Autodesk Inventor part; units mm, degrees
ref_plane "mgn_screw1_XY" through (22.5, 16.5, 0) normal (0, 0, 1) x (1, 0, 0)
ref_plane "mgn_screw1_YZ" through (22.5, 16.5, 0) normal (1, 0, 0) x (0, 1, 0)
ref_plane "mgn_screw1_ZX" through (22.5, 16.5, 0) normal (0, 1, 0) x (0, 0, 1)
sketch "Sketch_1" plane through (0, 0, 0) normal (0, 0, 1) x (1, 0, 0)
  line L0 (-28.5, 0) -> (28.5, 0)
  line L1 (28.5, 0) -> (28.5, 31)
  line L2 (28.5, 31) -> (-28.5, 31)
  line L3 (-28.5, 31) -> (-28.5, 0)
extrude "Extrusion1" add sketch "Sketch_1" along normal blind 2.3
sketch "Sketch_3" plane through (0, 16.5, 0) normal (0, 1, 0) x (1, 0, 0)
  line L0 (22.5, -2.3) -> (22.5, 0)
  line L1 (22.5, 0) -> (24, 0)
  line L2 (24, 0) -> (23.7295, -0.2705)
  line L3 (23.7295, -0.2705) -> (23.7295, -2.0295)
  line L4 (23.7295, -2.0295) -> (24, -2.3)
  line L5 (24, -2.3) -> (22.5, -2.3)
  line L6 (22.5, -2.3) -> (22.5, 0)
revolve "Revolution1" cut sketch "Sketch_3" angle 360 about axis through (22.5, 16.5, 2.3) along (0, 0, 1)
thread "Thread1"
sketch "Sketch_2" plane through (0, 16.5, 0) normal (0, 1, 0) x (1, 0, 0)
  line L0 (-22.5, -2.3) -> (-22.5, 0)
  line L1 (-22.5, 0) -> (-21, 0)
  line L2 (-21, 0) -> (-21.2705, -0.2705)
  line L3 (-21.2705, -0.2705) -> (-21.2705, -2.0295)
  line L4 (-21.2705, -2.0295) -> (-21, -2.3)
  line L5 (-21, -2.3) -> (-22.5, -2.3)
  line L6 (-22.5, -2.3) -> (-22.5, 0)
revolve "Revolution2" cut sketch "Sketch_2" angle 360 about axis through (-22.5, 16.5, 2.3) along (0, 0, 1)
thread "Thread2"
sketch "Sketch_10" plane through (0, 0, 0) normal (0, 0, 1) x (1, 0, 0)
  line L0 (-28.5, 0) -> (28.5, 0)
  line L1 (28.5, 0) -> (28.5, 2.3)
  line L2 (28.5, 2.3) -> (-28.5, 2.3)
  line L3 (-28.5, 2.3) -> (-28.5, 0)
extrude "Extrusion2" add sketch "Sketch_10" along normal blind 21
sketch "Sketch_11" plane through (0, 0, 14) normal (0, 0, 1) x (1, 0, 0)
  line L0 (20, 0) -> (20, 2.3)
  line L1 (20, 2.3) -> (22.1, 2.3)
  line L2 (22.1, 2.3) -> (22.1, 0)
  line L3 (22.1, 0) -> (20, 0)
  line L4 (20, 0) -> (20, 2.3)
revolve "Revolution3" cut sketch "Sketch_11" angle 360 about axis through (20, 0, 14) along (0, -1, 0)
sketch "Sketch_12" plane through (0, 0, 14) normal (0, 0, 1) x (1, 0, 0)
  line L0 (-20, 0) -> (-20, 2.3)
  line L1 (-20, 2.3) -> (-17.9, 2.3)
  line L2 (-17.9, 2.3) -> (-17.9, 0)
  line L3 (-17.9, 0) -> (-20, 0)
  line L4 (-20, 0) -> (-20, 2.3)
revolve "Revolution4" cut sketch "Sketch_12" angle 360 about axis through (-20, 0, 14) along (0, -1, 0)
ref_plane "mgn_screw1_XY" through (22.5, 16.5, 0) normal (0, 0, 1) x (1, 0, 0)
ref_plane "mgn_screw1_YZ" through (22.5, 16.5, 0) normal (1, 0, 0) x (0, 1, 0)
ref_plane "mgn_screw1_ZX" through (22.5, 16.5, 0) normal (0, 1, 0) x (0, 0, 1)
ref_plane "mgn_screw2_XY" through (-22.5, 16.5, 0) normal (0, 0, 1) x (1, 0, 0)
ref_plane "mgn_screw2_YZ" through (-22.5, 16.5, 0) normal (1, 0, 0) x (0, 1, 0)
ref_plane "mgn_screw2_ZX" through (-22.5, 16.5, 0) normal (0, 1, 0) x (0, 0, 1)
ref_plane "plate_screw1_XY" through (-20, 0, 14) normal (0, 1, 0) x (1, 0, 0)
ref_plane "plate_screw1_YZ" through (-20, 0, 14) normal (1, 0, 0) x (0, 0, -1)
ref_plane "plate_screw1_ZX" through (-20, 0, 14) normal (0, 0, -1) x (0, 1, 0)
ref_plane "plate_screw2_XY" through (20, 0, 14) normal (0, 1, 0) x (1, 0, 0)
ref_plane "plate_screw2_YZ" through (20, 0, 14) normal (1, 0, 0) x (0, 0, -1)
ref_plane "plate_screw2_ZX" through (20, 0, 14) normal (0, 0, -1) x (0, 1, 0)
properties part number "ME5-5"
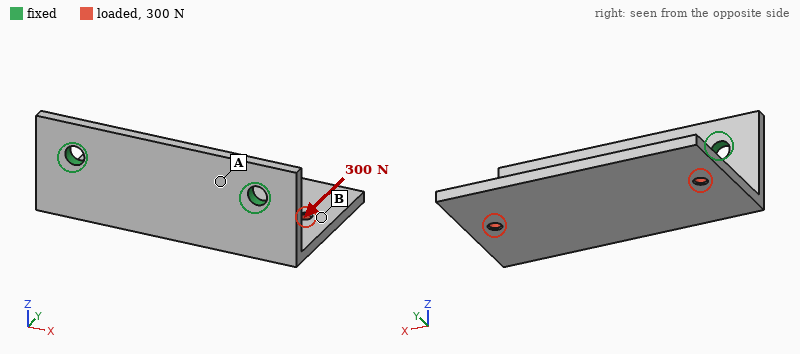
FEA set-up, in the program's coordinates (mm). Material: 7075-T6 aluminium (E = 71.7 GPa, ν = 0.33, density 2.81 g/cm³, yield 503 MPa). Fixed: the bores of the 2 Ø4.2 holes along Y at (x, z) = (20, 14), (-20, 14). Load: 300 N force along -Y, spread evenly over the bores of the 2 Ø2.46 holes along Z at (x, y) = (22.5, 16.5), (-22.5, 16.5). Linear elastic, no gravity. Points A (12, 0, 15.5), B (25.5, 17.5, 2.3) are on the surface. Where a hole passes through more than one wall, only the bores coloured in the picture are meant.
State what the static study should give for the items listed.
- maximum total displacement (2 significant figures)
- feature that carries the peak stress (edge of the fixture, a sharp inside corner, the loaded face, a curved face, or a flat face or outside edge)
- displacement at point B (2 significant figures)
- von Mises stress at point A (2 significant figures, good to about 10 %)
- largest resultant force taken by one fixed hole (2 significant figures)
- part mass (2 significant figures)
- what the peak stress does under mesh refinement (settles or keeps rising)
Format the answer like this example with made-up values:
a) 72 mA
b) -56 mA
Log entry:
a) 0.21 mm
b) edge of the fixture
c) 0.12 mm
d) 27 MPa
e) 150 N
f) 18 g
g) keeps rising
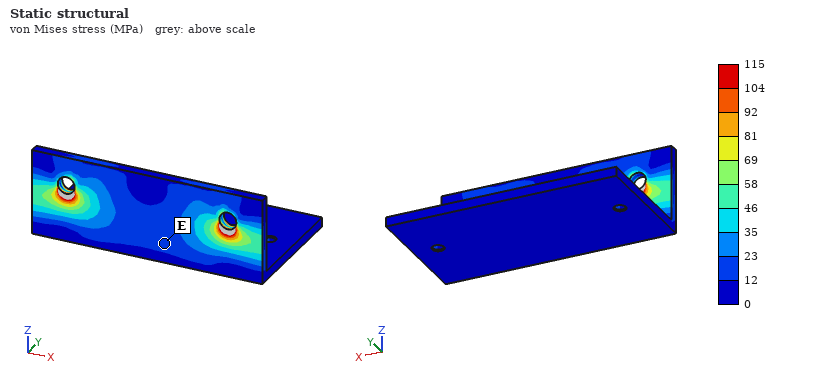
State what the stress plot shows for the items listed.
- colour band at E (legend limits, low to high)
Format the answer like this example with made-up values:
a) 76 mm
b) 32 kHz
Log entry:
a) 12 to 23 MPa
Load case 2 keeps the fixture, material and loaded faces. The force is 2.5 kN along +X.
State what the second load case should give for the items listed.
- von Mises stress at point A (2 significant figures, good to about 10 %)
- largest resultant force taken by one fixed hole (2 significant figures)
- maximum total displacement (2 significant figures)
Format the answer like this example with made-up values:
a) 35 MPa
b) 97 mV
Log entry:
a) 49 MPa
b) 1.7 kN
c) 0.66 mm
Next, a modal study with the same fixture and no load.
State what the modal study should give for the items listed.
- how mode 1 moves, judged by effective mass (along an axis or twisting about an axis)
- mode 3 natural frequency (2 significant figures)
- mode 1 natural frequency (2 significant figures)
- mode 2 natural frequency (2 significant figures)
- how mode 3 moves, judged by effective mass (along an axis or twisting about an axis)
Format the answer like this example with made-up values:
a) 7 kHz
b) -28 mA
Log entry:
a) along Z
b) 4300 Hz
c) 1200 Hz
d) 2500 Hz
e) along X
